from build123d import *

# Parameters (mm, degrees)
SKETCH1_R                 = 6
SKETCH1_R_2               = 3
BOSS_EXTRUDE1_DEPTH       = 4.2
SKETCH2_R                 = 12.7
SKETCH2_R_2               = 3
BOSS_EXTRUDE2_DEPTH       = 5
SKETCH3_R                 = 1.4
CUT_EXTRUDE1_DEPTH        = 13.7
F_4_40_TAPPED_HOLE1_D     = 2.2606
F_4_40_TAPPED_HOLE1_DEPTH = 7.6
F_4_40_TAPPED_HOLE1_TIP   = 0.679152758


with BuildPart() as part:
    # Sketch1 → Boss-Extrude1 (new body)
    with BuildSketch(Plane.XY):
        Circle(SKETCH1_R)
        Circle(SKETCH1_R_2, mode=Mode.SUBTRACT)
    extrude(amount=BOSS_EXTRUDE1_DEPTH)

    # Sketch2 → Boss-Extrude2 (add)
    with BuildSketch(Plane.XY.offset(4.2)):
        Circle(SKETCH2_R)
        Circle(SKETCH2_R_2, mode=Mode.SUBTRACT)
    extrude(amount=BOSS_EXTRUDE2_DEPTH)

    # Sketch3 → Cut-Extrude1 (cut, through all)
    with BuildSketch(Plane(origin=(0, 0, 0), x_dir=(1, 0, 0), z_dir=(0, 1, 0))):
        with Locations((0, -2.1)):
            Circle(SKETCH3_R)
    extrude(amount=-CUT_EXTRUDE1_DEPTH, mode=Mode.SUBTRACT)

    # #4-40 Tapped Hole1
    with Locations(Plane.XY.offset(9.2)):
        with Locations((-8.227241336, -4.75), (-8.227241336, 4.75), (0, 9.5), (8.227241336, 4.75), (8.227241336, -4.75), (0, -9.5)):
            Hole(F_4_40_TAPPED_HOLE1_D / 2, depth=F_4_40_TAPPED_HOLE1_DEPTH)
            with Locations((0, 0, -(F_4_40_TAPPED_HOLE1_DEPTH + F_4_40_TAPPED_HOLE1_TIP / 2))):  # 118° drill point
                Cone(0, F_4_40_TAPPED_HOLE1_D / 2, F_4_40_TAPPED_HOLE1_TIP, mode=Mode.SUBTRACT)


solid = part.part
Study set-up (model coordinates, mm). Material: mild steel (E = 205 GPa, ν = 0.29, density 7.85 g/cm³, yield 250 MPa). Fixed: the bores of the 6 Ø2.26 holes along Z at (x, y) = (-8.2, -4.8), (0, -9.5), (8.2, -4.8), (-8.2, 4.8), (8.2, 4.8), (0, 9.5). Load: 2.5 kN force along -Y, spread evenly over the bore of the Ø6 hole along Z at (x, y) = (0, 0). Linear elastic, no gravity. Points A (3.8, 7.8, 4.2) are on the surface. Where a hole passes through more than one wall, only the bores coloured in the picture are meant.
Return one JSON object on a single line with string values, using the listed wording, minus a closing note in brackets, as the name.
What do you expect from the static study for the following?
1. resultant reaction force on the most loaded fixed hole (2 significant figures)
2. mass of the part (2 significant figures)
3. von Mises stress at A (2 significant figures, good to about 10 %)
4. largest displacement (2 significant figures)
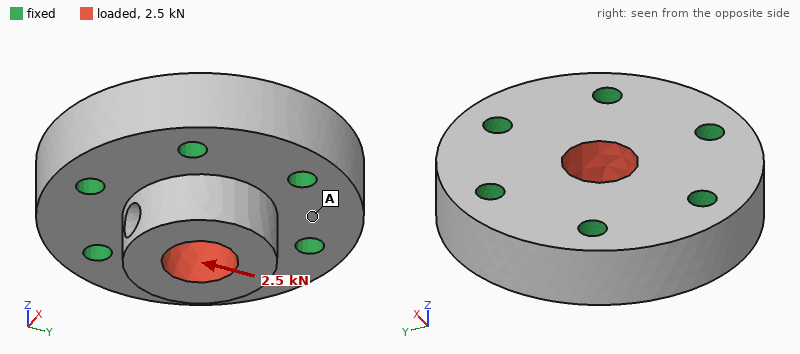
{"resultant reaction force on the most loaded fixed hole": "670 N", "mass of the part": "20 g", "von Mises stress at A": "7.9 MPa", "largest displacement": "1.9 µm"}
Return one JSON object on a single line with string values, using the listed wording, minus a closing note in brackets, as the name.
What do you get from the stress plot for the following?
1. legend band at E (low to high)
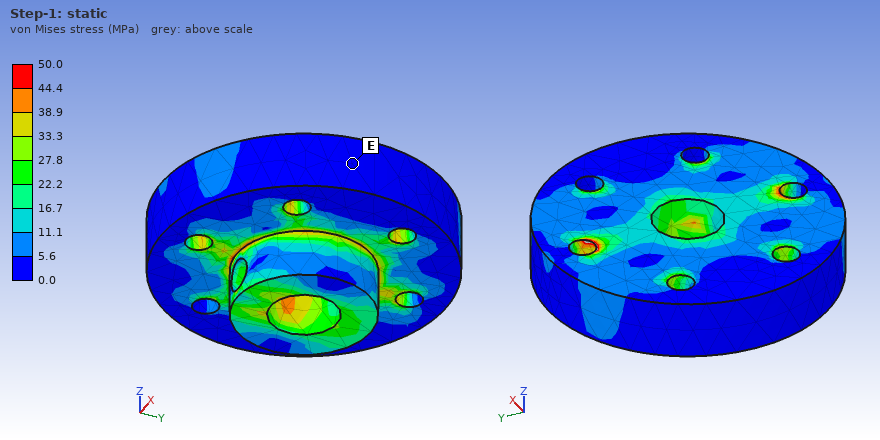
{"legend band at E": "0.0 to 5.6 MPa"}
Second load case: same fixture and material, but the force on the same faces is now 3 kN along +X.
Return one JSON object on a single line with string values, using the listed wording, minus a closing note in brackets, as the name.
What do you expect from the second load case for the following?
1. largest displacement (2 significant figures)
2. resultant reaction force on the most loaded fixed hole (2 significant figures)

{"largest displacement": "2.4 µm", "resultant reaction force on the most loaded fixed hole": "710 N"}
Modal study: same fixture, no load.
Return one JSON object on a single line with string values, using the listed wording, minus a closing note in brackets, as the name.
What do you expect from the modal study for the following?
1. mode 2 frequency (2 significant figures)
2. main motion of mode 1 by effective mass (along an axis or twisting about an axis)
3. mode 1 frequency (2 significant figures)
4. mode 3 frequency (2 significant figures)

{"mode 2 frequency": "90 kHz", "main motion of mode 1 by effective mass": "along Z", "mode 1 frequency": "84 kHz", "mode 3 frequency": "92 kHz"}
